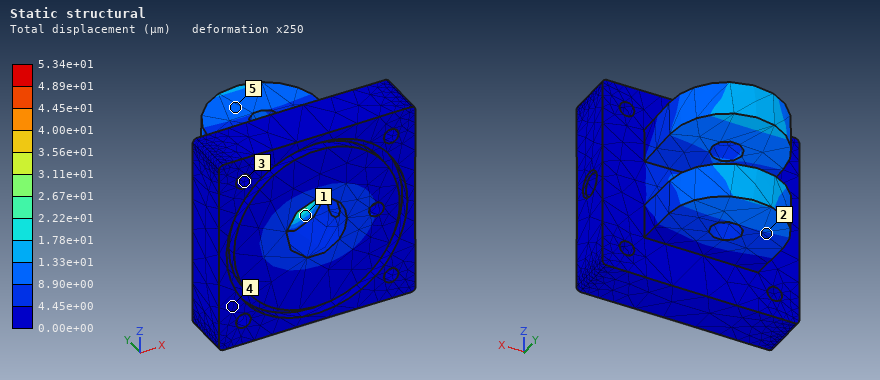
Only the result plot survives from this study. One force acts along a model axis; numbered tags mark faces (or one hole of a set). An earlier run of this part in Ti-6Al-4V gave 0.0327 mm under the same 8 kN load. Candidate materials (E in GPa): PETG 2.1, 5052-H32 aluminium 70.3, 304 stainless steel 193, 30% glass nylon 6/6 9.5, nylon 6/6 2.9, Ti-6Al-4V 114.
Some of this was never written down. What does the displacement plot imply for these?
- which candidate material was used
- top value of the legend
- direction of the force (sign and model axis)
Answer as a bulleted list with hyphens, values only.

- 5052-H32 aluminium
- 5.34e+01 µm
- +Y
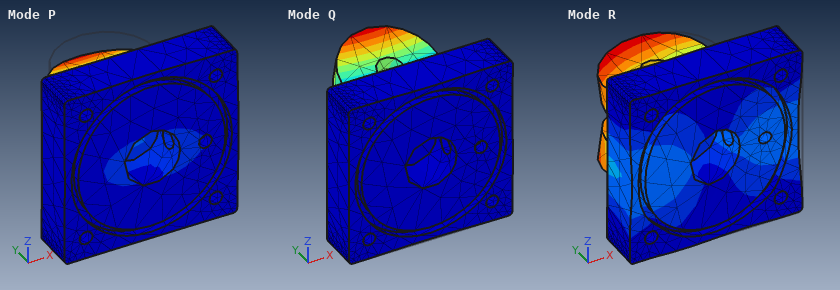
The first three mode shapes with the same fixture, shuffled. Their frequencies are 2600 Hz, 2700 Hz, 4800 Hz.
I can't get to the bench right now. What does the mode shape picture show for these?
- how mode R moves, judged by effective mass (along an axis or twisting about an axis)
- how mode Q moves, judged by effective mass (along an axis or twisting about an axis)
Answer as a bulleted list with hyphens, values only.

- along X
- along Z
